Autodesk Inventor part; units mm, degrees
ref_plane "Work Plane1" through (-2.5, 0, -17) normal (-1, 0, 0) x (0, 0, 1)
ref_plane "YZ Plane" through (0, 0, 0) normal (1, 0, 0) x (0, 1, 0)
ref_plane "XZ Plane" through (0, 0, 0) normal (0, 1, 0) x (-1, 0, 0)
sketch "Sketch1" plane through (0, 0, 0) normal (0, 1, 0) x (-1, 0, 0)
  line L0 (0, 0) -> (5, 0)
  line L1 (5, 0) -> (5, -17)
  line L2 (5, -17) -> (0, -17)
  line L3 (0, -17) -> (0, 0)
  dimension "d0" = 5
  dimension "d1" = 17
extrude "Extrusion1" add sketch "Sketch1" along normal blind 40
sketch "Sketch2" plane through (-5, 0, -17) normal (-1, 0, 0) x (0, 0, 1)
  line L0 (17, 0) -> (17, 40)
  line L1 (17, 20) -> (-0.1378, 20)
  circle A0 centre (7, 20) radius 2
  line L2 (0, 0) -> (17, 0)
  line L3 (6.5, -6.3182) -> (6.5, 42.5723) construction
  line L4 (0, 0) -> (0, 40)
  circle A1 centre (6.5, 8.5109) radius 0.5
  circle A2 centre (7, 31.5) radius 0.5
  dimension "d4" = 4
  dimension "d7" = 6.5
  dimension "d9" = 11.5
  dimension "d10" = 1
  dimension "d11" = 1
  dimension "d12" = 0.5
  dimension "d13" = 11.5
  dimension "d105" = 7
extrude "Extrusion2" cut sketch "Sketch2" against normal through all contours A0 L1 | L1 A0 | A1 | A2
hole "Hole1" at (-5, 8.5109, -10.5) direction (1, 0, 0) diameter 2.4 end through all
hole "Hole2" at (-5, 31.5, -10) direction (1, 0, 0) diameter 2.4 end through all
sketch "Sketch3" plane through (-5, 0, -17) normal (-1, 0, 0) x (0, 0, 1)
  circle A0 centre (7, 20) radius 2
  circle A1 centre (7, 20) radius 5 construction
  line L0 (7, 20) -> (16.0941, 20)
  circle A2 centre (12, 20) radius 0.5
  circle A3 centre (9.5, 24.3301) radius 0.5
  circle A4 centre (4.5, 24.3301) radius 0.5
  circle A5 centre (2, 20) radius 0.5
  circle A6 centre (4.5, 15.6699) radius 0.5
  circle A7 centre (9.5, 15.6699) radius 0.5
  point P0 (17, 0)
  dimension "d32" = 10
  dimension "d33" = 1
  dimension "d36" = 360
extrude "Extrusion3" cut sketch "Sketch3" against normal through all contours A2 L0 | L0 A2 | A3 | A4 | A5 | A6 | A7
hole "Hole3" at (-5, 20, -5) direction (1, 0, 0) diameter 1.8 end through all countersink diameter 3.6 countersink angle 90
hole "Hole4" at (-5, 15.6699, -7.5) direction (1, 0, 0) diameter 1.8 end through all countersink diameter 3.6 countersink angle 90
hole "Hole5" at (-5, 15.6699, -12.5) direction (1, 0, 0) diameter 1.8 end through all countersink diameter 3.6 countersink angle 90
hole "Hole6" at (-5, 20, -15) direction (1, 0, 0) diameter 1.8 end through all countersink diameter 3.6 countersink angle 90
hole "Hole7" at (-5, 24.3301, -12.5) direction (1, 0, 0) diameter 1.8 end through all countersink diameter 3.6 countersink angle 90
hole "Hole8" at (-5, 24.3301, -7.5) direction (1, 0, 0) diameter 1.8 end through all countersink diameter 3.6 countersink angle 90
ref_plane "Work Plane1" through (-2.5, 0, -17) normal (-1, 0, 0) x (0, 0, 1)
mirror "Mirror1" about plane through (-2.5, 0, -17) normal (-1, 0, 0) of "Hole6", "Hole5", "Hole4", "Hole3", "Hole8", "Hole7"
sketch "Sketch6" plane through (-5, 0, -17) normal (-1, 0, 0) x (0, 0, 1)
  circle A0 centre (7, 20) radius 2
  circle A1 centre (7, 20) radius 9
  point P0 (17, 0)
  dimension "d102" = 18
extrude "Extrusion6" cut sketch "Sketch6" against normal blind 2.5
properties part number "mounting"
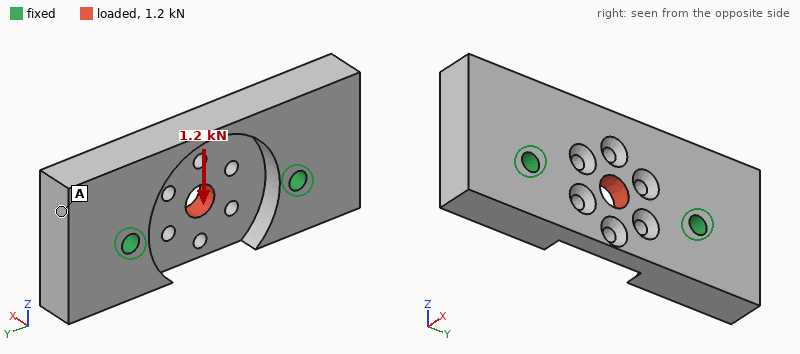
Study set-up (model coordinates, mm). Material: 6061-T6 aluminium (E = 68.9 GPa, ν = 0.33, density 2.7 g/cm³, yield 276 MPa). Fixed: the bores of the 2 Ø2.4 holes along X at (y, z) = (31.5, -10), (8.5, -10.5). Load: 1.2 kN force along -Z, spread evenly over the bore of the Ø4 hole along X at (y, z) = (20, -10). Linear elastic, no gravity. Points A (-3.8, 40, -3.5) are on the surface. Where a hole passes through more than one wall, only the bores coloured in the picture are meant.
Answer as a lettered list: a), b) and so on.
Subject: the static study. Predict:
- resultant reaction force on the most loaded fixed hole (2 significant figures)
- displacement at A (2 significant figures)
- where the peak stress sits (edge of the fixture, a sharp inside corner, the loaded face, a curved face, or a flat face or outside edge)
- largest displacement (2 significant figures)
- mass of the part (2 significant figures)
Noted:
a) 620 N
b) 3.6 µm
c) a curved face
d) 13 µm
e) 7.2 g
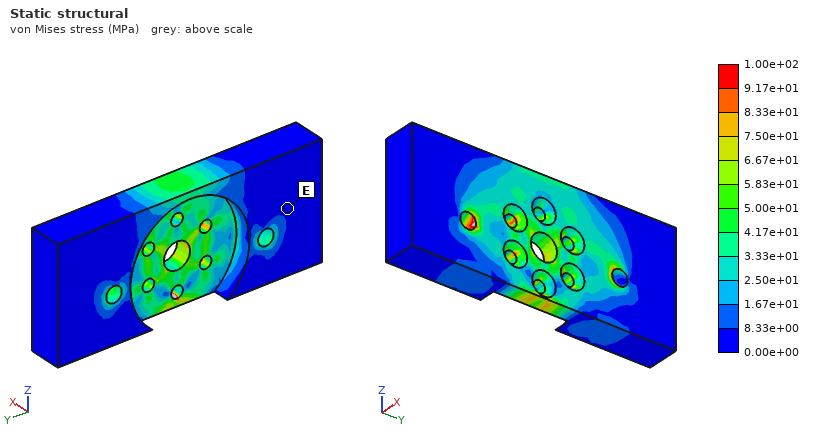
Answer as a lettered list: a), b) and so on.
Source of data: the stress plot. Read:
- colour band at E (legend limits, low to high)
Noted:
a) 0.00e+00 to 8.33e+00 MPa
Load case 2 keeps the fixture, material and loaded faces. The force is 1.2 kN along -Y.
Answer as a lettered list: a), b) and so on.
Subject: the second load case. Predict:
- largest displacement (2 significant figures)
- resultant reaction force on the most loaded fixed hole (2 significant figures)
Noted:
a) 5.2 µm
b) 610 N
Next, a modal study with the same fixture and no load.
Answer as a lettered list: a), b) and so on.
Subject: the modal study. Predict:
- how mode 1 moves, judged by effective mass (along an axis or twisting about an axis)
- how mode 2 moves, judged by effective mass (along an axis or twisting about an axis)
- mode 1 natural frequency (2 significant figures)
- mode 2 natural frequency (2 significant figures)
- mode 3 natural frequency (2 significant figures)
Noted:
a) along X
b) twisting about Z
c) 23 kHz
d) 26 kHz
e) 28 kHz
